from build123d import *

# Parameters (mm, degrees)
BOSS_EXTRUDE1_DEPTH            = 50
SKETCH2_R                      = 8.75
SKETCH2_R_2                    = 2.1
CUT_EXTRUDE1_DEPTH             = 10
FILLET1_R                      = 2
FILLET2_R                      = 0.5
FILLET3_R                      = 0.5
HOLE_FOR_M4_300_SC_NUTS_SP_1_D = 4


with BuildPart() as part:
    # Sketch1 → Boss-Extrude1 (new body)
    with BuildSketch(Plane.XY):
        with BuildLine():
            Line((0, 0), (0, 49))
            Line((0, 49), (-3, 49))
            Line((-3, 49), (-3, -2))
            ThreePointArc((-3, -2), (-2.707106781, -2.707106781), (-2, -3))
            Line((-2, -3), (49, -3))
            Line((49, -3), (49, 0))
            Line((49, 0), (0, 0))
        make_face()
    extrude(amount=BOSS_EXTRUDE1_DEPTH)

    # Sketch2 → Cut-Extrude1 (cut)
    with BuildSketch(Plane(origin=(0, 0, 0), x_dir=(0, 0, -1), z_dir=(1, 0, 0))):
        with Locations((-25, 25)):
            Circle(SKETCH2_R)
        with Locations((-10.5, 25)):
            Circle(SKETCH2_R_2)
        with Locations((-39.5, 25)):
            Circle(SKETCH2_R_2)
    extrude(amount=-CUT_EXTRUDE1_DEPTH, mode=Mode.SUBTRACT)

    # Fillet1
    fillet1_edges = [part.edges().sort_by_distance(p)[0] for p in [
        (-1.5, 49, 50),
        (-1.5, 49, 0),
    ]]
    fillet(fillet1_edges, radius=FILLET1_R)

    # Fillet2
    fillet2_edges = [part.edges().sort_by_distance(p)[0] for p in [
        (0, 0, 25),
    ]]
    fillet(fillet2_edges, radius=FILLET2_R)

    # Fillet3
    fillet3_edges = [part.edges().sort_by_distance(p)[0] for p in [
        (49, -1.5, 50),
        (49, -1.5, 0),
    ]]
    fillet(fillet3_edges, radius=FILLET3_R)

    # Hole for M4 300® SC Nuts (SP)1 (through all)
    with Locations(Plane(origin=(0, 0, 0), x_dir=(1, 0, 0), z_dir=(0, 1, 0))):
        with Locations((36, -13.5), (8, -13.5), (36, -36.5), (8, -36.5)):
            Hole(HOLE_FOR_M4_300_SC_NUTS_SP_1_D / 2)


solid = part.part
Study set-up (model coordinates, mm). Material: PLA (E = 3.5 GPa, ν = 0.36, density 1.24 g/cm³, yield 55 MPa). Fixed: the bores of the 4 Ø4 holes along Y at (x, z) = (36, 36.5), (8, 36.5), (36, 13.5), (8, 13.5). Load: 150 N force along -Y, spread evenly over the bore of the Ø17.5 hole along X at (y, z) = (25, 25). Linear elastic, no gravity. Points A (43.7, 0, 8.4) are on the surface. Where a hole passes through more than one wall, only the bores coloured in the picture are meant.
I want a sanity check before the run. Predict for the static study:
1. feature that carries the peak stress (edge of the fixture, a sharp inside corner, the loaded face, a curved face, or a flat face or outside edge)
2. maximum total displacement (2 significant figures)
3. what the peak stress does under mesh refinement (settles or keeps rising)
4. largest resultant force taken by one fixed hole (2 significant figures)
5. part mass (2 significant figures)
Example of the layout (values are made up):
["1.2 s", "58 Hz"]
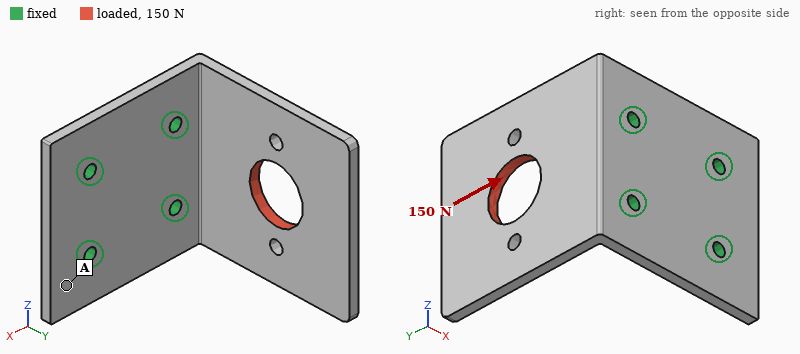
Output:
["edge of the fixture", "0.87 mm", "keeps rising", "80 N", "18 g"]
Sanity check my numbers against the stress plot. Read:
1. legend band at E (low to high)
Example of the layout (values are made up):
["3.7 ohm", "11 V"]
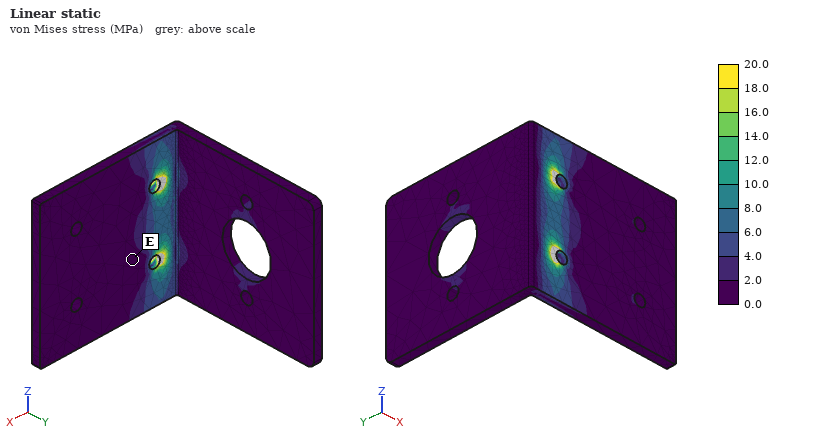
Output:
["0.0 to 2.0 MPa"]
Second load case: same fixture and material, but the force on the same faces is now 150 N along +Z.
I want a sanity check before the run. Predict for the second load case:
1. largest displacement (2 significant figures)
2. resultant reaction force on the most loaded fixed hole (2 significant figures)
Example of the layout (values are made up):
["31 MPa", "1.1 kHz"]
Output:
["0.85 mm", "170 N"]
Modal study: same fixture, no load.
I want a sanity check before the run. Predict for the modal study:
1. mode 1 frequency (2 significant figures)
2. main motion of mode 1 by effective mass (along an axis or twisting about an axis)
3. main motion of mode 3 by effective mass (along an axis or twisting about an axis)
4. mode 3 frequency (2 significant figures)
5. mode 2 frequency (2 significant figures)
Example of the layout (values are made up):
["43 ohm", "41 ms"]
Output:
["260 Hz", "along X", "along Z", "980 Hz", "630 Hz"]
